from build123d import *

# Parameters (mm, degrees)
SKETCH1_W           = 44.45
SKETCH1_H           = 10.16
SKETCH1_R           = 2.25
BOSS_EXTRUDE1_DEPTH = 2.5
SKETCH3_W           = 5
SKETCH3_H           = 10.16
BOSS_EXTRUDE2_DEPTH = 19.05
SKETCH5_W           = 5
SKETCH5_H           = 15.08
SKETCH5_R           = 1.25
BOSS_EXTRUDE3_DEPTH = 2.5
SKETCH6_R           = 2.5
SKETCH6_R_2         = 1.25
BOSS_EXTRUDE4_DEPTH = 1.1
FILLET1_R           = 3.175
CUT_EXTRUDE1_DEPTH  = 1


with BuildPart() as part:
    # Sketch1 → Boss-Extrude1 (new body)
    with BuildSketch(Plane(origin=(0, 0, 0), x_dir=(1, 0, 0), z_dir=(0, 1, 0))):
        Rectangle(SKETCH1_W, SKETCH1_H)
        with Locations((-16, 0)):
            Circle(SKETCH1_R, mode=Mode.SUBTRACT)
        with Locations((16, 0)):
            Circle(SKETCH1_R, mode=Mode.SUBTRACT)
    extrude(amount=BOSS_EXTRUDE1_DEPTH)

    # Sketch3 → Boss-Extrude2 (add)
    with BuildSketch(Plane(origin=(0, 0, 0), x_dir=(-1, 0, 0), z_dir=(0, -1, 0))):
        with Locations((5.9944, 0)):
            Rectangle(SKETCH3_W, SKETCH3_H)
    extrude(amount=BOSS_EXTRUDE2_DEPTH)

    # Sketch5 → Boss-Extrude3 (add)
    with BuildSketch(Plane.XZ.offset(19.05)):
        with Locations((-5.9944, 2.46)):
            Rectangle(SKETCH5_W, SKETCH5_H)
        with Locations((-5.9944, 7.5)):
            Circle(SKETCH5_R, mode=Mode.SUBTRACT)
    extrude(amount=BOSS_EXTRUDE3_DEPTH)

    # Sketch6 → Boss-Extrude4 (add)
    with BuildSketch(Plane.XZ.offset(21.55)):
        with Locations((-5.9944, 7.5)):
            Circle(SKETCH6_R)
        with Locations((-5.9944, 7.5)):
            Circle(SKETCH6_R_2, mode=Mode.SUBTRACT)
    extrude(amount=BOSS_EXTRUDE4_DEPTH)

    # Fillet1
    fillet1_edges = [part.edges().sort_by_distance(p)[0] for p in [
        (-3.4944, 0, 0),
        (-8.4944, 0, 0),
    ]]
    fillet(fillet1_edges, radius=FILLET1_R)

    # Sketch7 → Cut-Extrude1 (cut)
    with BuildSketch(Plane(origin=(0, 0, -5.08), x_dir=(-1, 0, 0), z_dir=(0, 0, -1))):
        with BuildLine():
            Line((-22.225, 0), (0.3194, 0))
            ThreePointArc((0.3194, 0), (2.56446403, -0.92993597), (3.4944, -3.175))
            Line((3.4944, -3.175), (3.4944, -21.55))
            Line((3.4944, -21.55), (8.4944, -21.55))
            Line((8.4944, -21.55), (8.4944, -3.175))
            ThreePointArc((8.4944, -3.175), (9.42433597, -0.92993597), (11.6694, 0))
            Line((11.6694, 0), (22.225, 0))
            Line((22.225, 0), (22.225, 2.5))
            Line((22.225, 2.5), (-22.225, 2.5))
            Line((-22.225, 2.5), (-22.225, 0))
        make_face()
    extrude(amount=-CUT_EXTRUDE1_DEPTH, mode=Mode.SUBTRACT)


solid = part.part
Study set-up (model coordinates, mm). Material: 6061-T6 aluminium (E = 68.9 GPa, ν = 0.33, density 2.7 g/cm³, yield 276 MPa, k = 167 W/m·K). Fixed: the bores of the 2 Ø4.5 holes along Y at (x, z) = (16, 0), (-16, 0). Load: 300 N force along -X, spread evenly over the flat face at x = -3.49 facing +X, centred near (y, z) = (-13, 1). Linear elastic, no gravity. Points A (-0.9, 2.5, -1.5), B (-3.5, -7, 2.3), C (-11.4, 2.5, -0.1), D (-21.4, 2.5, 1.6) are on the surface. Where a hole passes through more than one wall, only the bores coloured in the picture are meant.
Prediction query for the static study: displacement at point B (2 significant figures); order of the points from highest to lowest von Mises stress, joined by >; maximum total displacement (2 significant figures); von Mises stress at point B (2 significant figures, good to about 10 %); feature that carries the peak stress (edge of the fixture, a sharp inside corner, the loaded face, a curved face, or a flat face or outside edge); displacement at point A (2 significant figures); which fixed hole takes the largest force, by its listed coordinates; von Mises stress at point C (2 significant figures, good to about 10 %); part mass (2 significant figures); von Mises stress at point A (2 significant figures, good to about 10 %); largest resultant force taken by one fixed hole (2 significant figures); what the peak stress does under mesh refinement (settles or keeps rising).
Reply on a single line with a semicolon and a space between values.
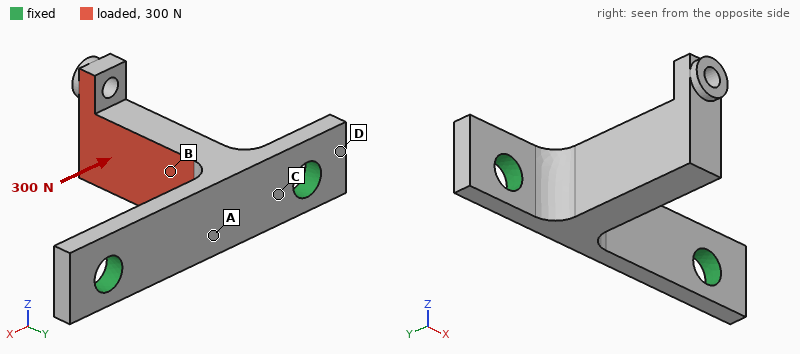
0.074 mm; A > C > B > D; 0.21 mm; 51 MPa; edge of the fixture; 0.051 mm; (-16, 0); 83 MPa; 5.5 g; 130 MPa; 260 N; keeps rising
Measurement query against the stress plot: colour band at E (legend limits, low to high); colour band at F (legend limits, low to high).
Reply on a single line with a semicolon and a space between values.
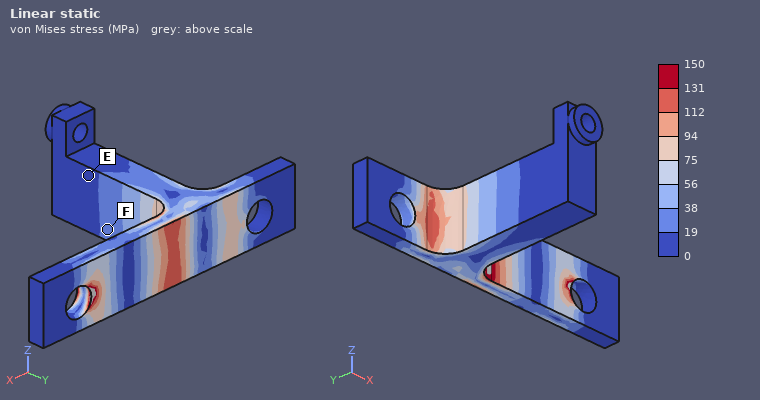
0 to 19 MPa; 19 to 38 MPa
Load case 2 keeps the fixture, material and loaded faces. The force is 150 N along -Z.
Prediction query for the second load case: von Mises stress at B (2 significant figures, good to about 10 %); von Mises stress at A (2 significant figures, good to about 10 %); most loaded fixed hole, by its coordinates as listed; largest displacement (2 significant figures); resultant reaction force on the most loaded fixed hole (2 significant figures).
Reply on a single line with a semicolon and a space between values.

14 MPa; 26 MPa; (-16, 0); 0.16 mm; 120 N
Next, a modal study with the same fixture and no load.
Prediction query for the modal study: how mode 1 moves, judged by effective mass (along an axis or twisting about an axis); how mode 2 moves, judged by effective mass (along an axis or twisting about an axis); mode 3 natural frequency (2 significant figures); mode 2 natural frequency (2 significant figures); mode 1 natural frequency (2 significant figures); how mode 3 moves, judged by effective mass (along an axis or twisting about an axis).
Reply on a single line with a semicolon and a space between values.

along Z; along X; 13 kHz; 4500 Hz; 3700 Hz; along Y
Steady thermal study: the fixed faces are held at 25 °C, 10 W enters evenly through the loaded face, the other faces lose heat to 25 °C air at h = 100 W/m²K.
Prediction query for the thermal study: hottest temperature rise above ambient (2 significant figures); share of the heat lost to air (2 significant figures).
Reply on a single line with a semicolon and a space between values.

26 K; 16 %
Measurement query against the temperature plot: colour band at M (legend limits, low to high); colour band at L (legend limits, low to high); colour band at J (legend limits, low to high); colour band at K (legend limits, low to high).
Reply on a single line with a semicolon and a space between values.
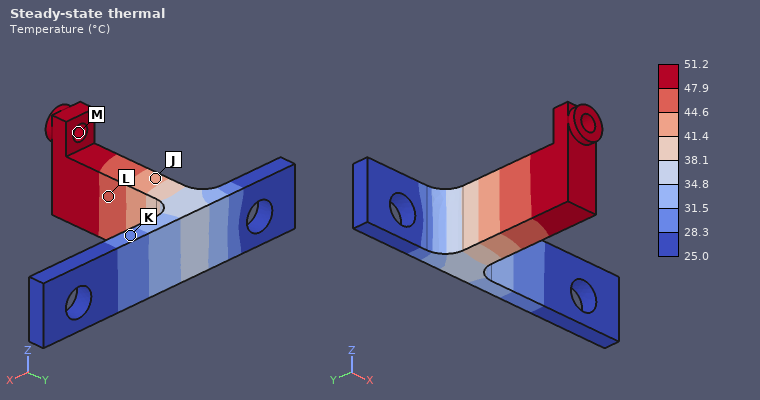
47.9 to 51.2 °C; 44.6 to 47.9 °C; 41.4 to 44.6 °C; 28.3 to 31.5 °C
